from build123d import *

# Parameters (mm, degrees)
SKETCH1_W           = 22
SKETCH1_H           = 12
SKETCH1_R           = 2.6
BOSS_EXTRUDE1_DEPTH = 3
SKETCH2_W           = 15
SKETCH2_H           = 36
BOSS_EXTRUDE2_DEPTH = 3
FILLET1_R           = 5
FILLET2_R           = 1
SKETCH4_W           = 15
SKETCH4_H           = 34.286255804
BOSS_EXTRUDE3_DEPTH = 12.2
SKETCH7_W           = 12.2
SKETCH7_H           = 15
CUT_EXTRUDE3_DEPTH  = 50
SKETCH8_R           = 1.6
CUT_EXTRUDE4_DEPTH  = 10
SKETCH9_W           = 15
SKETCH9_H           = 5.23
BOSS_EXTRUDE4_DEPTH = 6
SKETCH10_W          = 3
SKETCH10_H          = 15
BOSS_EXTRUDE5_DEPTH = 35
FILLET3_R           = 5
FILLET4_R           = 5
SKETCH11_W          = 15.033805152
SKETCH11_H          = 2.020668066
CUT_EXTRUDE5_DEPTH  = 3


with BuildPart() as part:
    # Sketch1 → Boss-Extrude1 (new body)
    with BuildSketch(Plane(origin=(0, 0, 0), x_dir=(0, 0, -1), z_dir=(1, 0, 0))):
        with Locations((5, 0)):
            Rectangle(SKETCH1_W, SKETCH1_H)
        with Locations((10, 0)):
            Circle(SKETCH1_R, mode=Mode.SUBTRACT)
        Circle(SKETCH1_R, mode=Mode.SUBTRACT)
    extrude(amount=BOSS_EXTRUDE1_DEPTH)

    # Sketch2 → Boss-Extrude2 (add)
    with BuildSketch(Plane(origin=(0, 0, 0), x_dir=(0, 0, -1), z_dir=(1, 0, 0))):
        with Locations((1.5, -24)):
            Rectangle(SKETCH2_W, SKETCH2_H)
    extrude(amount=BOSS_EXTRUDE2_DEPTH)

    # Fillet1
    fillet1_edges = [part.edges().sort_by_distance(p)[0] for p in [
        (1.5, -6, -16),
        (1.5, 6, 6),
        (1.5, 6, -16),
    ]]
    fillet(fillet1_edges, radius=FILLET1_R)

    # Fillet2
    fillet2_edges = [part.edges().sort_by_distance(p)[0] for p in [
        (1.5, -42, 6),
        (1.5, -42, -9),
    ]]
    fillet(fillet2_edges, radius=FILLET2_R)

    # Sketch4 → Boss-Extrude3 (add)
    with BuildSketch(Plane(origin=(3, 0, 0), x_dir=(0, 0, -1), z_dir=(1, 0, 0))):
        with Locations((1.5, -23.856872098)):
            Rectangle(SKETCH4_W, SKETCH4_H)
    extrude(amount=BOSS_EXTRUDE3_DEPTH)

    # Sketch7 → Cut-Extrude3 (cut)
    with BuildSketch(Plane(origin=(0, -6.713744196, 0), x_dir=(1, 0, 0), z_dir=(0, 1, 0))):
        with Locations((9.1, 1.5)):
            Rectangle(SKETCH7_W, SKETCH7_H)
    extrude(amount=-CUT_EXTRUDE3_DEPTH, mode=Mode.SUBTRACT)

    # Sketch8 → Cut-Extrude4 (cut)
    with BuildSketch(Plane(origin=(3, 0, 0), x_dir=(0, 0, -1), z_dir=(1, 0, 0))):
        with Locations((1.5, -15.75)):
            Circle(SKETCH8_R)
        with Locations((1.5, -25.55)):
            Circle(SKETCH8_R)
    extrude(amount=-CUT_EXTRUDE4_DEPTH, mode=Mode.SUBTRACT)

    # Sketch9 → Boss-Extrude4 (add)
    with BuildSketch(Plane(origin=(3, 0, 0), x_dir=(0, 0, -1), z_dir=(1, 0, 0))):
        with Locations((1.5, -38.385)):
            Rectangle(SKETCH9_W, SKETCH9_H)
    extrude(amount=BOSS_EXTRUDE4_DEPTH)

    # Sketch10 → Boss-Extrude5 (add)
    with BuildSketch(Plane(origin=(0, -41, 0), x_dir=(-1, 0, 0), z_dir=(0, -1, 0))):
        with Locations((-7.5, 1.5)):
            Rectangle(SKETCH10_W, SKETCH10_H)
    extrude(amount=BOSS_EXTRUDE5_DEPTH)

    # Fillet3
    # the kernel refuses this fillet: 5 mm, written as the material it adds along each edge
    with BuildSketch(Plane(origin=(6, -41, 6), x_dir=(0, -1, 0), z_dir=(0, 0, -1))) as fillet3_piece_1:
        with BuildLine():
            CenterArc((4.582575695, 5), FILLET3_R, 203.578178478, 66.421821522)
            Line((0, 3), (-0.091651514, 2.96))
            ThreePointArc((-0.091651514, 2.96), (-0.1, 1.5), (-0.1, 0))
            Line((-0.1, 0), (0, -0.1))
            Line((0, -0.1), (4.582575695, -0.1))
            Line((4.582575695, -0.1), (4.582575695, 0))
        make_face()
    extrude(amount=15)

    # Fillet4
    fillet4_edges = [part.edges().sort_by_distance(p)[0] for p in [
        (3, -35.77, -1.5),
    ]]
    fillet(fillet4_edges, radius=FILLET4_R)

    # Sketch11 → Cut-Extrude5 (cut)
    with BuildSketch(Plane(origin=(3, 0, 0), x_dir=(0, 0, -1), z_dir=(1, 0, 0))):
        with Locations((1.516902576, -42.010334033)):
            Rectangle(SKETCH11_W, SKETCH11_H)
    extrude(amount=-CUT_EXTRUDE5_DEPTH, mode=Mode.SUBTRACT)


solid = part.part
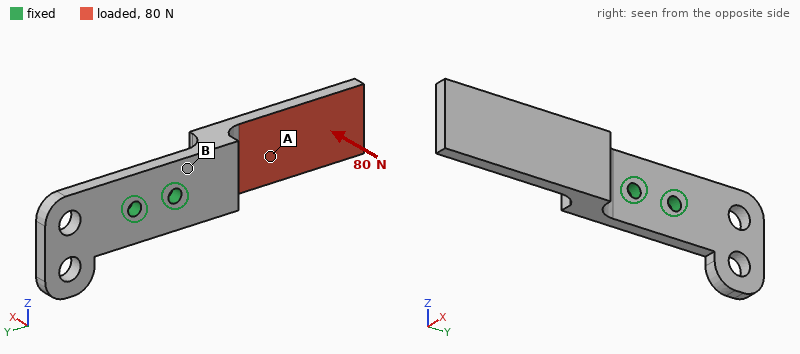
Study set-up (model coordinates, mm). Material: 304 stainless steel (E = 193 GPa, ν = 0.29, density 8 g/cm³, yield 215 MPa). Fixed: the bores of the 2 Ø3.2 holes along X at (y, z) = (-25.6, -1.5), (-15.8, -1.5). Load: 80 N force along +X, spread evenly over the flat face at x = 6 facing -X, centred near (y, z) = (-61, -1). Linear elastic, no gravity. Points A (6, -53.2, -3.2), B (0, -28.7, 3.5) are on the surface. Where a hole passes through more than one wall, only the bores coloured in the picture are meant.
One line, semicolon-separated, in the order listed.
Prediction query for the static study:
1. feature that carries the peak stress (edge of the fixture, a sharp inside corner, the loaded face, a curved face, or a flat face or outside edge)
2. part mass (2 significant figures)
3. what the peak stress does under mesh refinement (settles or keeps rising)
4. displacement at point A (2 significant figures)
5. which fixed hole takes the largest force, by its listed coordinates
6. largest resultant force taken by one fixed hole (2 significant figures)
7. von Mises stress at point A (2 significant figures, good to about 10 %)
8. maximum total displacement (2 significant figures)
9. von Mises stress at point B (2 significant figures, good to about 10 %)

edge of the fixture; 35 g; keeps rising; 0.087 mm; (-25.6, -1.5); 160 N; 30 MPa; 0.22 mm; 93 MPa
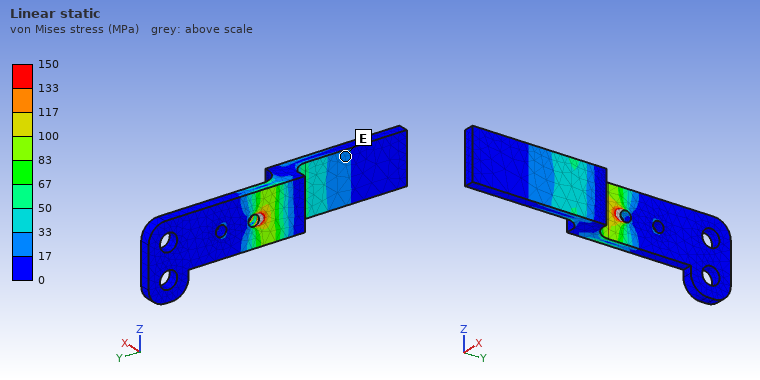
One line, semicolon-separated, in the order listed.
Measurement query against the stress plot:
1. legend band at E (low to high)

17 to 33 MPa
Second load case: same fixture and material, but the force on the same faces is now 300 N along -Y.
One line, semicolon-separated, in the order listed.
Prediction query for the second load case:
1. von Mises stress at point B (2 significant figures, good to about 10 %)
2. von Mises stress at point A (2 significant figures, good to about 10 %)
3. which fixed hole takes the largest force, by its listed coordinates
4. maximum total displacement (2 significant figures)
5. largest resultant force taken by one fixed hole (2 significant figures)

45 MPa; 20 MPa; (-25.6, -1.5); 52 µm; 250 N
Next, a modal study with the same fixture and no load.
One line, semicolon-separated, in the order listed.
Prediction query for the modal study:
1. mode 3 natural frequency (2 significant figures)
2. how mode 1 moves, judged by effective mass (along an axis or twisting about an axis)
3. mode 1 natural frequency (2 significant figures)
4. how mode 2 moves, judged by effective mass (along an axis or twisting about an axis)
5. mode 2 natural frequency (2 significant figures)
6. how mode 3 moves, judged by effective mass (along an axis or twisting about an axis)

4600 Hz; along X; 1100 Hz; along Z; 3400 Hz; along X
